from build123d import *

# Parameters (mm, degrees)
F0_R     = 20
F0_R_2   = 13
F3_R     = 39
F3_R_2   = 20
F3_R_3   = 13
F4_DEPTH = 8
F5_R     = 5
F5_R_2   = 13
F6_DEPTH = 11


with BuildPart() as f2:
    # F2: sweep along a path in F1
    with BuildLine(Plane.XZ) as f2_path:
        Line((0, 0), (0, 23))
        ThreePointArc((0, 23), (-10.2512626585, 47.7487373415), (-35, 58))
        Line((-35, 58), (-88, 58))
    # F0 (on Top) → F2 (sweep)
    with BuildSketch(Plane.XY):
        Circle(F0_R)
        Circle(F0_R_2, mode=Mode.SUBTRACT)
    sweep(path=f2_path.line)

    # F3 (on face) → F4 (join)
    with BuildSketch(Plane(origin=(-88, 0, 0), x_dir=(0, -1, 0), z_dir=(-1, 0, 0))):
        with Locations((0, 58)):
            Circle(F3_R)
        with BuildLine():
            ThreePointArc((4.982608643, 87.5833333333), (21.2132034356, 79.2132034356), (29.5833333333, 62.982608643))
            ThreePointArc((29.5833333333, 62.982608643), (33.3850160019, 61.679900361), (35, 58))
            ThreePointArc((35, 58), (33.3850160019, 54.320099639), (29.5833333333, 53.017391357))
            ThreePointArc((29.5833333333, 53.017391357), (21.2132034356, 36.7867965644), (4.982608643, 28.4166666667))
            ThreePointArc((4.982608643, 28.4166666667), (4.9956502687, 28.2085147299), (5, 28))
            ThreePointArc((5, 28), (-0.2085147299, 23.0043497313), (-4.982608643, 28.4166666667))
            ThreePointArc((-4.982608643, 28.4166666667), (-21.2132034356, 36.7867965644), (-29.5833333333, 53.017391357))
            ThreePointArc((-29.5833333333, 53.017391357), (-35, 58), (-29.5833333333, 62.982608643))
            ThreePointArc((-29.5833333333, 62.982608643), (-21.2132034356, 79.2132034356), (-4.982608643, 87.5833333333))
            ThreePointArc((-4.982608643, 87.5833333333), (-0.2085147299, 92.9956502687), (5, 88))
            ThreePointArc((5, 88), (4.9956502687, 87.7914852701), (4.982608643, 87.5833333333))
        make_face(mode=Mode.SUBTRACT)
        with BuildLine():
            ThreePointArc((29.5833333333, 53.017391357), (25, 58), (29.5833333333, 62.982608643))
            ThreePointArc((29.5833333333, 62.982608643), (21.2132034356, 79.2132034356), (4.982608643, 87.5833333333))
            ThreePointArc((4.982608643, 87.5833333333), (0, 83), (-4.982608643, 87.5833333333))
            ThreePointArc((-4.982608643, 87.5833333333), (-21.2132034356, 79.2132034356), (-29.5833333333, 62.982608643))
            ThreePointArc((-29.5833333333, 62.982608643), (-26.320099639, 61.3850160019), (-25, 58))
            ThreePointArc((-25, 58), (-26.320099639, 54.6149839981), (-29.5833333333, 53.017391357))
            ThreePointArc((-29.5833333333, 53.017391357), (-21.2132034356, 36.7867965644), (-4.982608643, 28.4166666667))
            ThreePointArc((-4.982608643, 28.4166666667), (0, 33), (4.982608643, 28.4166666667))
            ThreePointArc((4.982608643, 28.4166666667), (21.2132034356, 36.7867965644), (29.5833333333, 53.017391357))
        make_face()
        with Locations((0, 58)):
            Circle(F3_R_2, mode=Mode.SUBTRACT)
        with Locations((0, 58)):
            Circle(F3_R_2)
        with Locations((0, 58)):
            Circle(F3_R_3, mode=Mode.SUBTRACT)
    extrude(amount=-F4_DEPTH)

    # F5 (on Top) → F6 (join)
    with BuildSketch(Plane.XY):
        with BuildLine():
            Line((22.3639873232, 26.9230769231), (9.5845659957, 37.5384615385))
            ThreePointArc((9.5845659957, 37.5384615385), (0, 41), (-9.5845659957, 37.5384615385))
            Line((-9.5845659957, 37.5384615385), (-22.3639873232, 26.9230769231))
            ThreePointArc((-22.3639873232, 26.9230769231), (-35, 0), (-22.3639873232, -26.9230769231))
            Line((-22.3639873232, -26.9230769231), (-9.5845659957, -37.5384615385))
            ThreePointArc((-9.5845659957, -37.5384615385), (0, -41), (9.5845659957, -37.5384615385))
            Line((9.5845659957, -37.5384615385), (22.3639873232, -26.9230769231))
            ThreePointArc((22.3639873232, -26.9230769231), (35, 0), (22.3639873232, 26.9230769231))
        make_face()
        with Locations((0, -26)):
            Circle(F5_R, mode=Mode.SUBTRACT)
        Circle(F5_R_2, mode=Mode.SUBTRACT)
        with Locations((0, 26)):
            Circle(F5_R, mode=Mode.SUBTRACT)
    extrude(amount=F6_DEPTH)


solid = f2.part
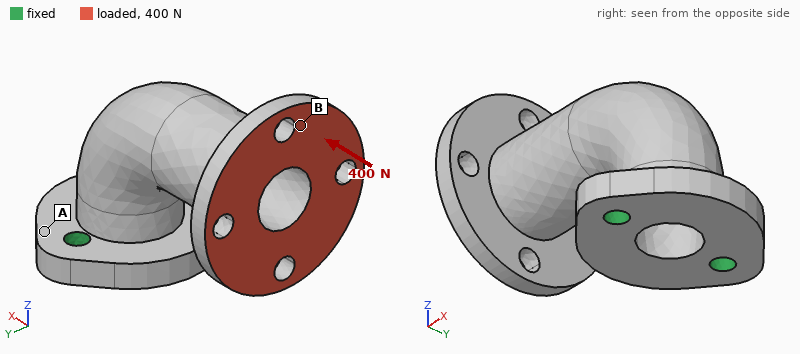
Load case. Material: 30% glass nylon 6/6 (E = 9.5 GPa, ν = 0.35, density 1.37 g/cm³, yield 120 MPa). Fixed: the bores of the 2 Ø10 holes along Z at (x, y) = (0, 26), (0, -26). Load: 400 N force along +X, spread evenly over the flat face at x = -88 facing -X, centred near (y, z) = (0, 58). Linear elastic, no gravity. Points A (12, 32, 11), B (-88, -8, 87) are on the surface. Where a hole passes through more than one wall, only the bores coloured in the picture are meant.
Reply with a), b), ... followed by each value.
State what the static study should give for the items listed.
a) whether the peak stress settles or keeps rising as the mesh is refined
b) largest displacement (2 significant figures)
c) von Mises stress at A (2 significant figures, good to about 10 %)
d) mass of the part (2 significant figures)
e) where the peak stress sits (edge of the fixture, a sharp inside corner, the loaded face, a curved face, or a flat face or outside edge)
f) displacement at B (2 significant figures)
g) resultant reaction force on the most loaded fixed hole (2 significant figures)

a) keeps rising
b) 0.32 mm
c) 4.2 MPa
d) 210 g
e) edge of the fixture
f) 0.30 mm
g) 200 N
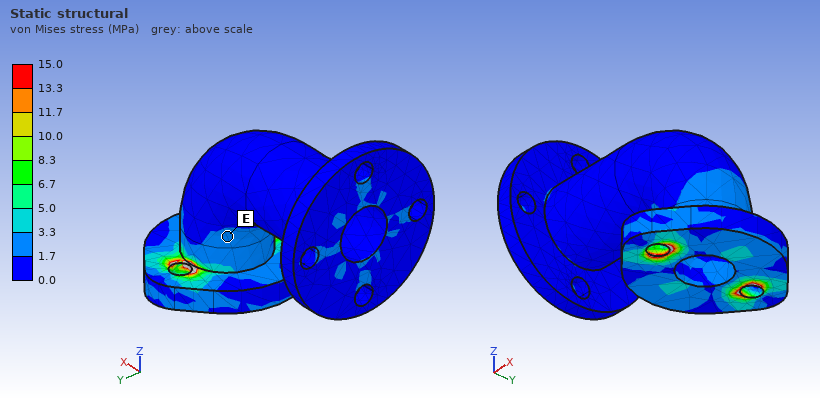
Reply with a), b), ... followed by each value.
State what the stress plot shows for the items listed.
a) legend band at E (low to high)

a) 1.7 to 3.3 MPa
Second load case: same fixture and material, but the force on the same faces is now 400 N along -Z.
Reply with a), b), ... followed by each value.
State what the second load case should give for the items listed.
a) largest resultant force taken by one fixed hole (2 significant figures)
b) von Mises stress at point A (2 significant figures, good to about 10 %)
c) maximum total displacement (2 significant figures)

a) 250 N
b) 7.0 MPa
c) 0.72 mm
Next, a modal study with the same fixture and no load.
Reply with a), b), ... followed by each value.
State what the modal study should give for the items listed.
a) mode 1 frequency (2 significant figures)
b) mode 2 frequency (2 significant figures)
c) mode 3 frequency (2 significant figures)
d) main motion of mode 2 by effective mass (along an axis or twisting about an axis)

a) 470 Hz
b) 690 Hz
c) 1700 Hz
d) along Y
